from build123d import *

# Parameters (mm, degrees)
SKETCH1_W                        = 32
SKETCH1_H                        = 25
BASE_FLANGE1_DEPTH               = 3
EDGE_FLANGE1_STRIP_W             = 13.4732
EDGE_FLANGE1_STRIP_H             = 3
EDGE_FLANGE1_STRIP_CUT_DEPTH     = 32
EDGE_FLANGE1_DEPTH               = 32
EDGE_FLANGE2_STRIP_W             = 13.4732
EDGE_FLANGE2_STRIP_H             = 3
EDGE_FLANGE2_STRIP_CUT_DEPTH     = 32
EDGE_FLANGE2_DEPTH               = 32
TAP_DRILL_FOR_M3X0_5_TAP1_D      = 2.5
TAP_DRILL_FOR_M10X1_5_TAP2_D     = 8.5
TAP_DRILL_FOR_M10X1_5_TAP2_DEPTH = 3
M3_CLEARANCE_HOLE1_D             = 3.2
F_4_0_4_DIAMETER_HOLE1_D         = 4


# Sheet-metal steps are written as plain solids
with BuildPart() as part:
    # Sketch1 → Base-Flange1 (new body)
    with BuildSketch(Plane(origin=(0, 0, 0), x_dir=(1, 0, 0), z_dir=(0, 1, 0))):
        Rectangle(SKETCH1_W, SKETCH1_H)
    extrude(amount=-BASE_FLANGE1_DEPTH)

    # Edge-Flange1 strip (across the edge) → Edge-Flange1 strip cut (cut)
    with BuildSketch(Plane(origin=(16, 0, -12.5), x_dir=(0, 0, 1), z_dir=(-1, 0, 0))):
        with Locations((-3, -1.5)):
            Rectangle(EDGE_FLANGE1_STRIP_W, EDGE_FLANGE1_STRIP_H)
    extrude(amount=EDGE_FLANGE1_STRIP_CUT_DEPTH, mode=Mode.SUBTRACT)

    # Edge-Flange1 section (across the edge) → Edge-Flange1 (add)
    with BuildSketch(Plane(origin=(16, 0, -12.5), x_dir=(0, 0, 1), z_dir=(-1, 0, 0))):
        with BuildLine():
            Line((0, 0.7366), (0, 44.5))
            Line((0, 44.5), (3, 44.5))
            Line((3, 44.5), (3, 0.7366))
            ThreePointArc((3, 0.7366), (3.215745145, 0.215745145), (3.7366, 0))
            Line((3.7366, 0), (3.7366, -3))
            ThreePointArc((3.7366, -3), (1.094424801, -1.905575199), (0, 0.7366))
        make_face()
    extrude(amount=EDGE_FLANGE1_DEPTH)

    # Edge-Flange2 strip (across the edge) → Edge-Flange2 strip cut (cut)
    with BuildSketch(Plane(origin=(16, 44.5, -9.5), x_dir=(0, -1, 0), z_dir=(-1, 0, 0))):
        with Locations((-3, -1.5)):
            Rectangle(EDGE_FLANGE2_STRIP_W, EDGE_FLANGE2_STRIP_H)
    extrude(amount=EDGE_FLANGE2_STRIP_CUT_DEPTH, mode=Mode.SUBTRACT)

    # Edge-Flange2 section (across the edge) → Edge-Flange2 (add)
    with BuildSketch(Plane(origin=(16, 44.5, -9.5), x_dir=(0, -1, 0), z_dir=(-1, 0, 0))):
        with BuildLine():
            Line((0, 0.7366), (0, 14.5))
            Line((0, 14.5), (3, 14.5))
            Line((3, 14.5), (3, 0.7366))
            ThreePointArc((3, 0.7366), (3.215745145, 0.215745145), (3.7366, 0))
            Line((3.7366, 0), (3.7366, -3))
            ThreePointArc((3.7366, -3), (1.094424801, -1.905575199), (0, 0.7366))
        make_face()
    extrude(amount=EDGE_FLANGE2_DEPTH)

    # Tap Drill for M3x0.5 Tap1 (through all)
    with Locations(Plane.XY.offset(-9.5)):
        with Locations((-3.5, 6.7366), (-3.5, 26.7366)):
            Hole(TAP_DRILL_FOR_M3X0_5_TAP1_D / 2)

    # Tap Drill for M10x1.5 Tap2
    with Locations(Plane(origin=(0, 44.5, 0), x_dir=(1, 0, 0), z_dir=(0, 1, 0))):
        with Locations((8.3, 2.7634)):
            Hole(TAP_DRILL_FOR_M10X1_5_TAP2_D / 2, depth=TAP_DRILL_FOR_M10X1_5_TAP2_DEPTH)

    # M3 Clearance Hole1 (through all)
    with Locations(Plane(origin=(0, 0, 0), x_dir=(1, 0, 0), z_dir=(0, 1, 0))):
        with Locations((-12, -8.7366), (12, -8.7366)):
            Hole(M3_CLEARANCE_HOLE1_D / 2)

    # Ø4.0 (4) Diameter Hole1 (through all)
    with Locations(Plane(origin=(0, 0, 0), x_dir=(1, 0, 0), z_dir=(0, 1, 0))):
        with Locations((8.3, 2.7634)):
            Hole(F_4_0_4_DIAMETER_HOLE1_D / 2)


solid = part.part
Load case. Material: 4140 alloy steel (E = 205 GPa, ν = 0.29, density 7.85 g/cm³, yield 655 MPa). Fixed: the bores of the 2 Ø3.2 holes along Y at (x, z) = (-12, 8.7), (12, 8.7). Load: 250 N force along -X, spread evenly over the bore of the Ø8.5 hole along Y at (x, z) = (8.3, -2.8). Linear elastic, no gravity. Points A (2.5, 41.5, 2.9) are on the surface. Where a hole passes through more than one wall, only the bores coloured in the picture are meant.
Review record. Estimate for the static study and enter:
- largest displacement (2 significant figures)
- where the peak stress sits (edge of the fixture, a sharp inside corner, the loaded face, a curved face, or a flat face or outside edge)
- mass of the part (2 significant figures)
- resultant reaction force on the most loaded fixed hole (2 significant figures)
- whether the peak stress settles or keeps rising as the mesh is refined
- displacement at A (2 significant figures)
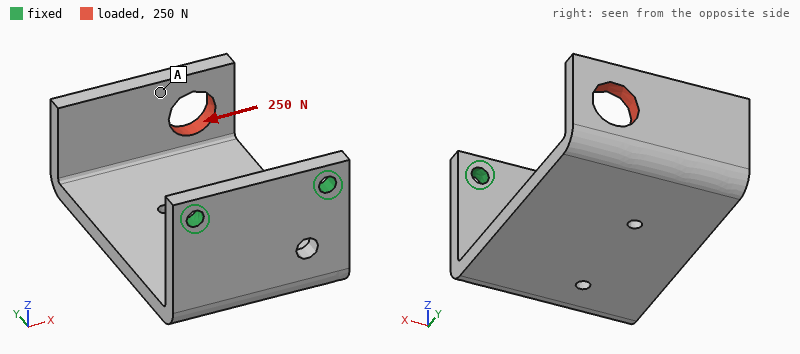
0.35 mm
edge of the fixture
60 g
480 N
keeps rising
0.30 mm
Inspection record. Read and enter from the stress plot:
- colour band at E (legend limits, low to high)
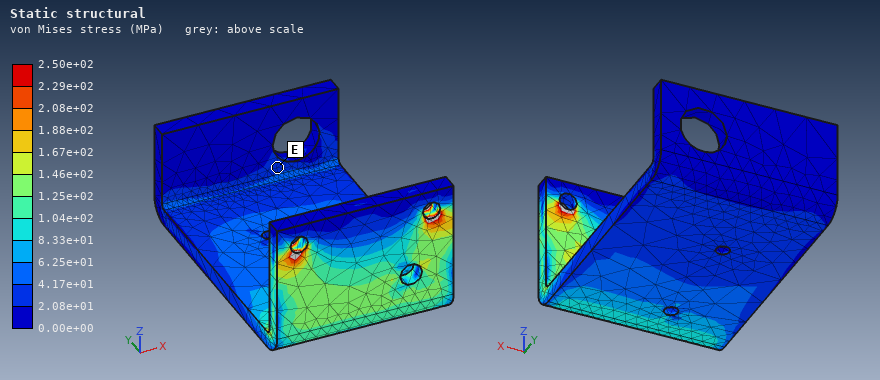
2.08e+01 to 4.17e+01 MPa
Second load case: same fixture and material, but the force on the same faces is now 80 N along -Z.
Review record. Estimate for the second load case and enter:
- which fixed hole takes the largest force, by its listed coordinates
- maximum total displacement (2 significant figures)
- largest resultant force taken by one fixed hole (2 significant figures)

(12, 8.7)
0.42 mm
71 N
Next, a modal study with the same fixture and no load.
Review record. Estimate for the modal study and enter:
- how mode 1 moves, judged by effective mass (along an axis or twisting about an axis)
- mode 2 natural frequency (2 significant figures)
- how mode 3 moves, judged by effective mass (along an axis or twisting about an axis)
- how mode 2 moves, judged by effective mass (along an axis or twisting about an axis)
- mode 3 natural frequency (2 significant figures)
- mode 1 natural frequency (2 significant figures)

along Z
1100 Hz
along Y
along X
2000 Hz
520 Hz
